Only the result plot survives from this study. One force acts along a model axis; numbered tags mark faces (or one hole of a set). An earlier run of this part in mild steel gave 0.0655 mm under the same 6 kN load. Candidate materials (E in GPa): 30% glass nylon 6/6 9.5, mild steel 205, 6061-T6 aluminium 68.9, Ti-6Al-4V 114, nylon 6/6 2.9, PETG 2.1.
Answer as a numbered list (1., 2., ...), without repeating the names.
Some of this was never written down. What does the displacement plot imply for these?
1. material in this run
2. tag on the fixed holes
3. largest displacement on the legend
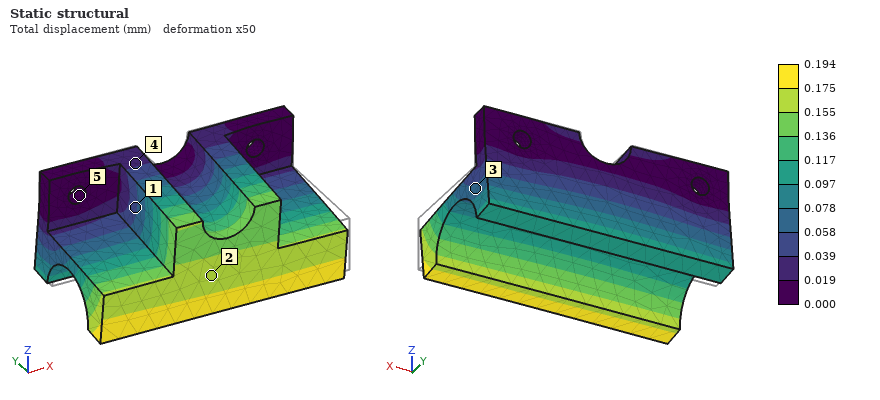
1. 6061-T6 aluminium
2. 5
3. 0.194 mm
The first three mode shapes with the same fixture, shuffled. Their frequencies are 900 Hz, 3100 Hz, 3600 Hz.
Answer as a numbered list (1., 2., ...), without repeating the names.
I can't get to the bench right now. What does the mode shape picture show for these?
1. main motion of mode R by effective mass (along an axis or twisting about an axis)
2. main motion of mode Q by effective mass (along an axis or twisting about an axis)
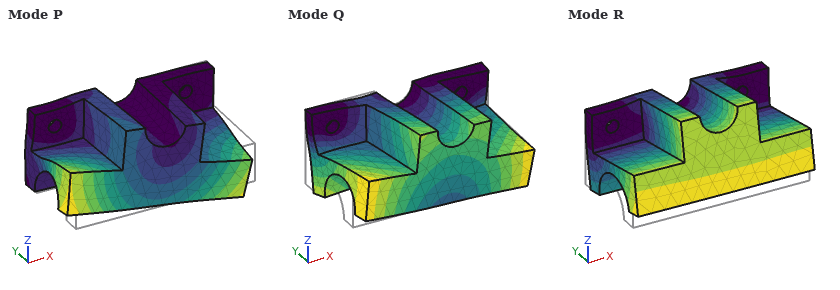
1. along Z
2. along X
